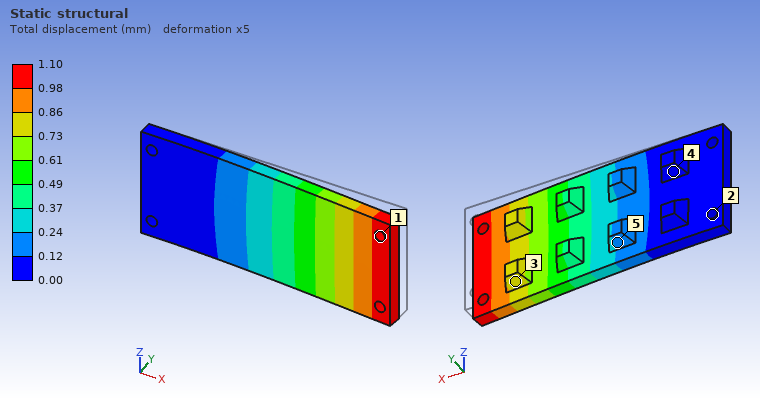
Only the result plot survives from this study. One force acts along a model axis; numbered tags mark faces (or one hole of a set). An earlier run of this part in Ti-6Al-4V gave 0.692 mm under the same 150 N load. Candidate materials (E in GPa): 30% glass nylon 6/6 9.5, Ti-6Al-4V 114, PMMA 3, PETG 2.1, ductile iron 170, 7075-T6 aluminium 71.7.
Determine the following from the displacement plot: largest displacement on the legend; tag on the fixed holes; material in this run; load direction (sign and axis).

1.10 mm
2
7075-T6 aluminium
-Y
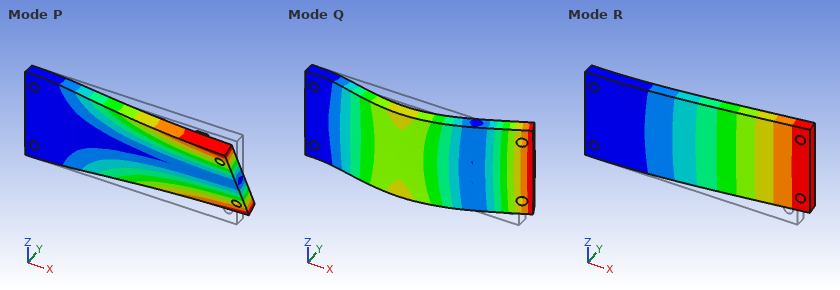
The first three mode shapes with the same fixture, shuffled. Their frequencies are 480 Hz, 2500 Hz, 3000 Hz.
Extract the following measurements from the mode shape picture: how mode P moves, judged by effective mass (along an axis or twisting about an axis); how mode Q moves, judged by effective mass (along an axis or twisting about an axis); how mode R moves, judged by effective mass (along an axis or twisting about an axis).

twisting about X
along Y
along Y
